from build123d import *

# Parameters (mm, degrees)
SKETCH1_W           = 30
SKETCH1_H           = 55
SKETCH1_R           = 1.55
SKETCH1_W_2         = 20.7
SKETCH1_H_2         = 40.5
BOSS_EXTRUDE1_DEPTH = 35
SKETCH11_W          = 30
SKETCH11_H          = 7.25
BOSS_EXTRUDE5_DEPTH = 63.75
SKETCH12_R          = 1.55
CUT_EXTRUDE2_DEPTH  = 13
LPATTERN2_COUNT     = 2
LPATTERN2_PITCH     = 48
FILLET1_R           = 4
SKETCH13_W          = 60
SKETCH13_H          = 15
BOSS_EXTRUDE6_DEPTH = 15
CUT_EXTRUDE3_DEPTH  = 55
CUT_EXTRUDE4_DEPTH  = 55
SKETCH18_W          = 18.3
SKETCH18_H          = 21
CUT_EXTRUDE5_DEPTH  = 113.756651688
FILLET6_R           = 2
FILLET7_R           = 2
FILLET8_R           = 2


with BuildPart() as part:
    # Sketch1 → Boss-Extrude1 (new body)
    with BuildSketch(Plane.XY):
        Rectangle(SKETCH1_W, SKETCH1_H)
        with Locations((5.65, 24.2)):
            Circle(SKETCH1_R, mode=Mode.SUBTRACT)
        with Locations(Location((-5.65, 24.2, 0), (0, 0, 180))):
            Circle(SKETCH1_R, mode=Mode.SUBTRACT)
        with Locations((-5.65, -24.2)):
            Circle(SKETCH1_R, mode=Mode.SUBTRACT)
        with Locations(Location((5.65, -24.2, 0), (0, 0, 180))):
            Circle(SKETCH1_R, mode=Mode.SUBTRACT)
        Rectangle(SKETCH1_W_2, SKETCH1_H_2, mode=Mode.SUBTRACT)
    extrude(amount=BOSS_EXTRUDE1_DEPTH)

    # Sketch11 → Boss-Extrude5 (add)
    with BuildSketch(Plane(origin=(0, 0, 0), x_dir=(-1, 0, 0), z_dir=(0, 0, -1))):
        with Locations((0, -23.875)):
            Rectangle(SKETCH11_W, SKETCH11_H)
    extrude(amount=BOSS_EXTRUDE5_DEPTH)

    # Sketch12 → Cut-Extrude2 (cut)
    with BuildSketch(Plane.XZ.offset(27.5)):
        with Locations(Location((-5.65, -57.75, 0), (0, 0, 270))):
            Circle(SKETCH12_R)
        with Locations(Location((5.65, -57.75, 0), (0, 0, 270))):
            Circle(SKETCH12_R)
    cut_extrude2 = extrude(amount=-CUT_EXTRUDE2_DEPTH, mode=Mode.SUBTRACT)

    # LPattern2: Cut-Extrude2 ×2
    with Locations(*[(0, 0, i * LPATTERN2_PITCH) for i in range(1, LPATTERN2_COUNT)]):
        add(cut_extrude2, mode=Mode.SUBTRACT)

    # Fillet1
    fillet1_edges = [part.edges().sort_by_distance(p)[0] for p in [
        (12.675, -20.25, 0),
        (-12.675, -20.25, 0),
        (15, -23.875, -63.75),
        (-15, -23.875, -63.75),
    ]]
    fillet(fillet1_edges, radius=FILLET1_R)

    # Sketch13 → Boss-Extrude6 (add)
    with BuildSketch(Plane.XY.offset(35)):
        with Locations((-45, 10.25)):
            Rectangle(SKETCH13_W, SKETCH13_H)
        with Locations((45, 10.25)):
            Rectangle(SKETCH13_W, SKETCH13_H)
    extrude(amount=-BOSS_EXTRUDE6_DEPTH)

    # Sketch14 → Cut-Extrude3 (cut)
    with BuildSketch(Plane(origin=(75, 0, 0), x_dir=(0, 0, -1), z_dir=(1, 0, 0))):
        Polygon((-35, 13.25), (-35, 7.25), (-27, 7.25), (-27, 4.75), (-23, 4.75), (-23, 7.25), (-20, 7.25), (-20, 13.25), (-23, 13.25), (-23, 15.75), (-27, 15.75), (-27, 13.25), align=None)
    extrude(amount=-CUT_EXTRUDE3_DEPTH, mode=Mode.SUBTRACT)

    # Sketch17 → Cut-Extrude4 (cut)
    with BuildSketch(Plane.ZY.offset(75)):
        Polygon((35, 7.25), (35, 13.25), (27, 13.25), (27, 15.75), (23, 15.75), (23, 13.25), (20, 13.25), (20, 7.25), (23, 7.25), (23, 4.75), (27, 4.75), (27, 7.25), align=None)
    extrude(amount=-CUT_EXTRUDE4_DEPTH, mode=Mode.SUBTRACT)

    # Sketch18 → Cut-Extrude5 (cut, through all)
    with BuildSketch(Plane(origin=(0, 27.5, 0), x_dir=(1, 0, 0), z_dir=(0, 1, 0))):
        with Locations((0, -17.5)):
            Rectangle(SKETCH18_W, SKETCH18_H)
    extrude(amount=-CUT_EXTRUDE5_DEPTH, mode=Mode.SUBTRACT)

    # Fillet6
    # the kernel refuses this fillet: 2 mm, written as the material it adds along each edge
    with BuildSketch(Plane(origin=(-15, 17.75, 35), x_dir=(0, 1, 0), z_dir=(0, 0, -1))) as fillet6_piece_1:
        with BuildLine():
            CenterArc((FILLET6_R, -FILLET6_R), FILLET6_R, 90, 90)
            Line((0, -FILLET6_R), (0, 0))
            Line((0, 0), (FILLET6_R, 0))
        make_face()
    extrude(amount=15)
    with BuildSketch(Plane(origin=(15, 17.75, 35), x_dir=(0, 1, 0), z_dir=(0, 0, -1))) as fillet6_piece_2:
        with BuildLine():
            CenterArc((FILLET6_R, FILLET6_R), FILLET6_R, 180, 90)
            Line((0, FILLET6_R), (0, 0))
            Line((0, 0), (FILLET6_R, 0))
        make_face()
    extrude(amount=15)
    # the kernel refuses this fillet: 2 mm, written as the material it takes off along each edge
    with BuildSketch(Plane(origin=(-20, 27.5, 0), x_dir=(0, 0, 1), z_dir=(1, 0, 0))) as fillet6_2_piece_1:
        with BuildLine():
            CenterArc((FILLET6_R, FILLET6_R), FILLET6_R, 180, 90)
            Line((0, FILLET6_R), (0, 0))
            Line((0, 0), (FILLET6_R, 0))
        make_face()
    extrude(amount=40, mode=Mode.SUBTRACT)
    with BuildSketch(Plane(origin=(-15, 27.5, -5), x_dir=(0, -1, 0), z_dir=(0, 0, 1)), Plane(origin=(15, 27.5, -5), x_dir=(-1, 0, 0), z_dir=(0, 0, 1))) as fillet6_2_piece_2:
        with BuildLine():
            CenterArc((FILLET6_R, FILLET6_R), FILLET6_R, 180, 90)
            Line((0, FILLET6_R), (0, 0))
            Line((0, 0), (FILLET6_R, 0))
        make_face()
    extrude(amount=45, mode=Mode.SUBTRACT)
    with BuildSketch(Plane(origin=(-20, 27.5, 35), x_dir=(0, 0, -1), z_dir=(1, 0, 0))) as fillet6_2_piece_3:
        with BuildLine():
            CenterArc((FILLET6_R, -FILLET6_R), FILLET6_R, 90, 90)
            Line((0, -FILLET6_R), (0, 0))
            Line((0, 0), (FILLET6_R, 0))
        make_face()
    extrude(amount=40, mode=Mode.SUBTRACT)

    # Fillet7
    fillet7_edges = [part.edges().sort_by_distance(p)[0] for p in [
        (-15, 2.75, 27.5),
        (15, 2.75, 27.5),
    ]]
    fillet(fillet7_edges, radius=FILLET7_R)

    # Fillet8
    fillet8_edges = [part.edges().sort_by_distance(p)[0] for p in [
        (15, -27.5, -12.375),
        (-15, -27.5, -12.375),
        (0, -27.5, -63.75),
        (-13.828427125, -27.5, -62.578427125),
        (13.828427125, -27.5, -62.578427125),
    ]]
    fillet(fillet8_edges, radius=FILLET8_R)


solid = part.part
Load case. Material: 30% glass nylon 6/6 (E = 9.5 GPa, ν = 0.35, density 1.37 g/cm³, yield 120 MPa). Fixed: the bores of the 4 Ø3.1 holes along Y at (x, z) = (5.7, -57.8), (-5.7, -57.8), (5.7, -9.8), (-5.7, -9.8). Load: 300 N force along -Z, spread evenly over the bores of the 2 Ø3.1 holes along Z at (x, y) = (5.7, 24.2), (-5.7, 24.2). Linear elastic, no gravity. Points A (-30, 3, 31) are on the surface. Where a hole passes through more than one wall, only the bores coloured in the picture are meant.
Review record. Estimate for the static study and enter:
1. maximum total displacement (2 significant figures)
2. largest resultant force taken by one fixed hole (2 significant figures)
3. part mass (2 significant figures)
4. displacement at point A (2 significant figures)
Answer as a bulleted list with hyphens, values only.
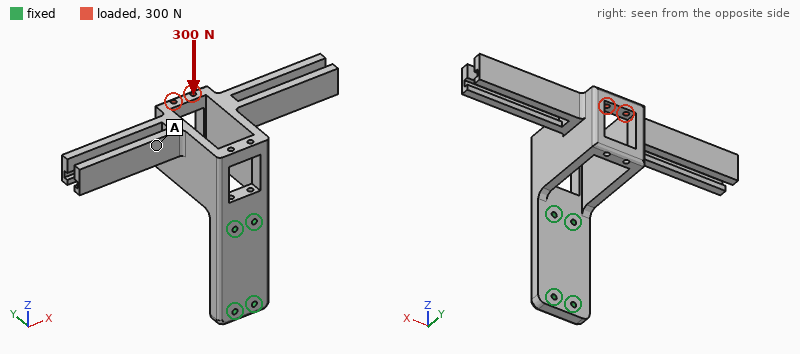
- 1.9 mm
- 130 N
- 69 g
- 1.2 mm
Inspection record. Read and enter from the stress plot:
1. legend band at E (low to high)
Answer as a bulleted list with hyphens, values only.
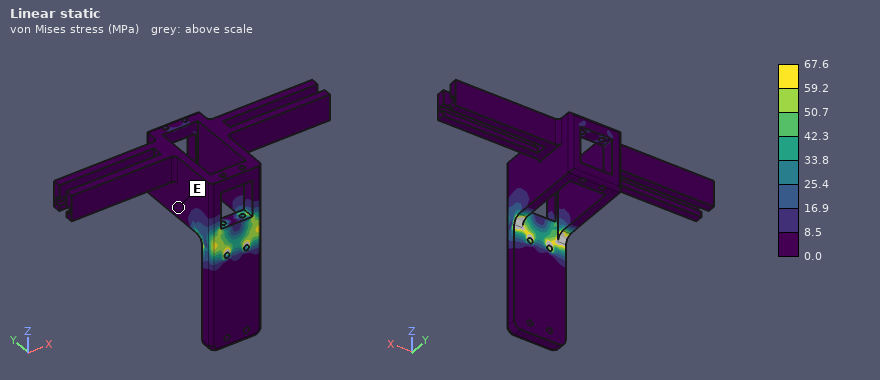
- 0.0 to 8.5 MPa
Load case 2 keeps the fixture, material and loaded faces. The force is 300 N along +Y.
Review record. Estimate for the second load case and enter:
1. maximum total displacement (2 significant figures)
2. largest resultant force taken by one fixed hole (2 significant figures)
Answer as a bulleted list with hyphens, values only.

- 1.3 mm
- 170 N
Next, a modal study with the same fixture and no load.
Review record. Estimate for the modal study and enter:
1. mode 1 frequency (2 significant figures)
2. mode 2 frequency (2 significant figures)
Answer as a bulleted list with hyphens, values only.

- 350 Hz
- 360 Hz
